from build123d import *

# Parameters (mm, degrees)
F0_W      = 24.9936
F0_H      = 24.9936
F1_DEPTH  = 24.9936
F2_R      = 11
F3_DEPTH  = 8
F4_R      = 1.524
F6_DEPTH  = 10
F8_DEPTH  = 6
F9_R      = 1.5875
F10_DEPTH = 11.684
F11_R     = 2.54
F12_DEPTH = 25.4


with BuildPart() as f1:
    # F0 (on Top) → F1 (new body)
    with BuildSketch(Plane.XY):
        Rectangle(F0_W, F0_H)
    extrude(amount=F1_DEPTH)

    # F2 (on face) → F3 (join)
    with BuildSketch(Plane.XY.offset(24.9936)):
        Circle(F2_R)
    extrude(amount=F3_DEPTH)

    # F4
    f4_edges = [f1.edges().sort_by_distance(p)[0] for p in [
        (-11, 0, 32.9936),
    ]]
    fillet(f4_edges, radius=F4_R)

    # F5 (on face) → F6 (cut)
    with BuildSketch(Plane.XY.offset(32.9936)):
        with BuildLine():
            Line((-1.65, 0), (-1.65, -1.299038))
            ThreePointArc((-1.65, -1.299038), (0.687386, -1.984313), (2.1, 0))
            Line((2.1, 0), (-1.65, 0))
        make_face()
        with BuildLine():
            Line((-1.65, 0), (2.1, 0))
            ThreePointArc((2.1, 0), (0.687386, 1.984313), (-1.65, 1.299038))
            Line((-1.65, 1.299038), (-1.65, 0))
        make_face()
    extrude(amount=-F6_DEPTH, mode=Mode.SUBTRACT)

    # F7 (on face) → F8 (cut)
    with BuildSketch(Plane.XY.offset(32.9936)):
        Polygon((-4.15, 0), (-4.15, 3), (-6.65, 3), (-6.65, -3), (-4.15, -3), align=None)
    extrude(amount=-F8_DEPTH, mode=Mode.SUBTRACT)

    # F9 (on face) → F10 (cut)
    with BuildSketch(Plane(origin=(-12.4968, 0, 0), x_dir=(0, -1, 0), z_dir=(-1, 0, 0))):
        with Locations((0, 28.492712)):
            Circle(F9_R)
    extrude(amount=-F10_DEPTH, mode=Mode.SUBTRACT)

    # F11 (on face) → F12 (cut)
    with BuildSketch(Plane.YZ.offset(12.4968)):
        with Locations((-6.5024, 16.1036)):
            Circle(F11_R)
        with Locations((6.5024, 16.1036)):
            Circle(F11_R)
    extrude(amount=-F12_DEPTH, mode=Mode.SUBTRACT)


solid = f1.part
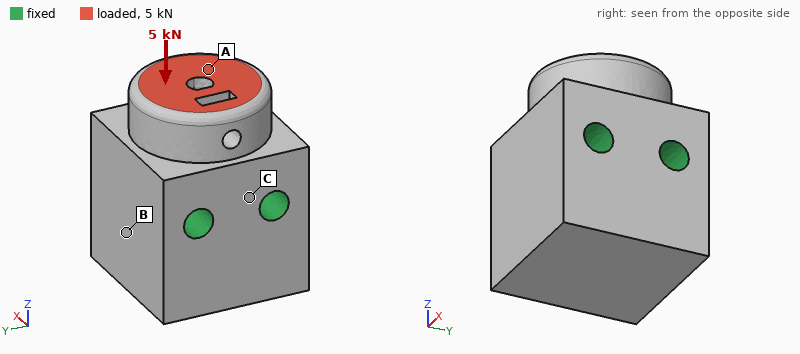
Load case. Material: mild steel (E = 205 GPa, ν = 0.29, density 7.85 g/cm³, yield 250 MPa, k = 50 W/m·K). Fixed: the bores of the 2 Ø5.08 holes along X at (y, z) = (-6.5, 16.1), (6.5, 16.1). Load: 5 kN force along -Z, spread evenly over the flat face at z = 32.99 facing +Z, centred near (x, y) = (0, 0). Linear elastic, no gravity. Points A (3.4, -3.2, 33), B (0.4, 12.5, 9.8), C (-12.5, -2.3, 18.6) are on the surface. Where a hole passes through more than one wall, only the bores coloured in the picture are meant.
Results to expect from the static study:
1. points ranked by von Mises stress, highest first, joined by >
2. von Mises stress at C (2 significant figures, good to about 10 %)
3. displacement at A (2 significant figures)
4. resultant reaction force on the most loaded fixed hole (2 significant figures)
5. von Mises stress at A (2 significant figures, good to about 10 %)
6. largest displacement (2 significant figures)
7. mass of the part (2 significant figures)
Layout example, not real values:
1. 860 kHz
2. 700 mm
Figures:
1. A > C > B
2. 4.6 MPa
3. 1.1 µm
4. 2.6 kN
5. 13 MPa
6. 1.5 µm
7. 140 g
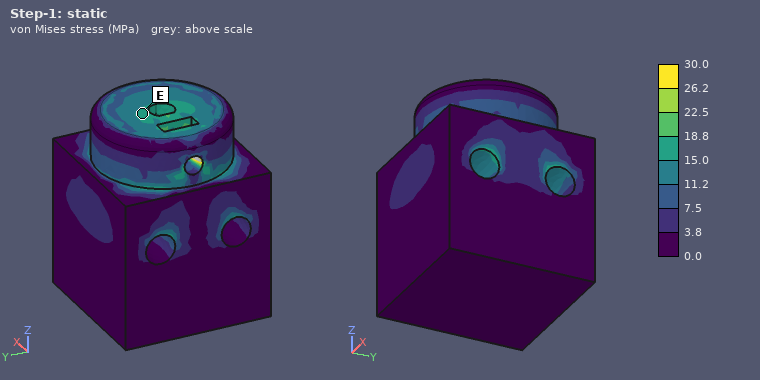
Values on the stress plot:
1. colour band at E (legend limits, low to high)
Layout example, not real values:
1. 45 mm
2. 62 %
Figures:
1. 15.0 to 18.8 MPa
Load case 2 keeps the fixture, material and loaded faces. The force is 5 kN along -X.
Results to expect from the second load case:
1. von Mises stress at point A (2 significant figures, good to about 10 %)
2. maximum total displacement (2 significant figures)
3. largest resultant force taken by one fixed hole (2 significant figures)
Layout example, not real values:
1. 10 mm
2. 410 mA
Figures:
1. 38 MPa
2. 5.7 µm
3. 2.5 kN
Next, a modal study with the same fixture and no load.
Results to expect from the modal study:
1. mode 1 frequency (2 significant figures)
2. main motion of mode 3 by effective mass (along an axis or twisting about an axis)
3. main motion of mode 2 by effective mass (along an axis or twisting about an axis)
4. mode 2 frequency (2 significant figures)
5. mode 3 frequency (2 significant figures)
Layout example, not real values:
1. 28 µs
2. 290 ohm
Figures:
1. 39 kHz
2. along Y
3. along X
4. 42 kHz
5. 46 kHz
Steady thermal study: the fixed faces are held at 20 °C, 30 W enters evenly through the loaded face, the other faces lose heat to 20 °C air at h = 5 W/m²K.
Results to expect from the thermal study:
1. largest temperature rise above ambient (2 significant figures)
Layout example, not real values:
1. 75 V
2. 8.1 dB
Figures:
1. 27 K
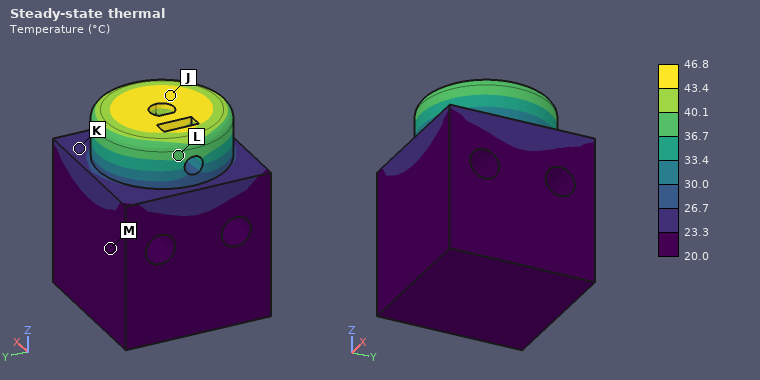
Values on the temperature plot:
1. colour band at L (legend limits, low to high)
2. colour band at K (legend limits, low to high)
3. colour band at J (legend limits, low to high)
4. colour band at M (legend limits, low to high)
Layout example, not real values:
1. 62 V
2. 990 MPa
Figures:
1. 36.7 to 40.1 °C
2. 23.3 to 26.7 °C
3. 43.4 to 46.8 °C
4. 20.0 to 23.3 °C
